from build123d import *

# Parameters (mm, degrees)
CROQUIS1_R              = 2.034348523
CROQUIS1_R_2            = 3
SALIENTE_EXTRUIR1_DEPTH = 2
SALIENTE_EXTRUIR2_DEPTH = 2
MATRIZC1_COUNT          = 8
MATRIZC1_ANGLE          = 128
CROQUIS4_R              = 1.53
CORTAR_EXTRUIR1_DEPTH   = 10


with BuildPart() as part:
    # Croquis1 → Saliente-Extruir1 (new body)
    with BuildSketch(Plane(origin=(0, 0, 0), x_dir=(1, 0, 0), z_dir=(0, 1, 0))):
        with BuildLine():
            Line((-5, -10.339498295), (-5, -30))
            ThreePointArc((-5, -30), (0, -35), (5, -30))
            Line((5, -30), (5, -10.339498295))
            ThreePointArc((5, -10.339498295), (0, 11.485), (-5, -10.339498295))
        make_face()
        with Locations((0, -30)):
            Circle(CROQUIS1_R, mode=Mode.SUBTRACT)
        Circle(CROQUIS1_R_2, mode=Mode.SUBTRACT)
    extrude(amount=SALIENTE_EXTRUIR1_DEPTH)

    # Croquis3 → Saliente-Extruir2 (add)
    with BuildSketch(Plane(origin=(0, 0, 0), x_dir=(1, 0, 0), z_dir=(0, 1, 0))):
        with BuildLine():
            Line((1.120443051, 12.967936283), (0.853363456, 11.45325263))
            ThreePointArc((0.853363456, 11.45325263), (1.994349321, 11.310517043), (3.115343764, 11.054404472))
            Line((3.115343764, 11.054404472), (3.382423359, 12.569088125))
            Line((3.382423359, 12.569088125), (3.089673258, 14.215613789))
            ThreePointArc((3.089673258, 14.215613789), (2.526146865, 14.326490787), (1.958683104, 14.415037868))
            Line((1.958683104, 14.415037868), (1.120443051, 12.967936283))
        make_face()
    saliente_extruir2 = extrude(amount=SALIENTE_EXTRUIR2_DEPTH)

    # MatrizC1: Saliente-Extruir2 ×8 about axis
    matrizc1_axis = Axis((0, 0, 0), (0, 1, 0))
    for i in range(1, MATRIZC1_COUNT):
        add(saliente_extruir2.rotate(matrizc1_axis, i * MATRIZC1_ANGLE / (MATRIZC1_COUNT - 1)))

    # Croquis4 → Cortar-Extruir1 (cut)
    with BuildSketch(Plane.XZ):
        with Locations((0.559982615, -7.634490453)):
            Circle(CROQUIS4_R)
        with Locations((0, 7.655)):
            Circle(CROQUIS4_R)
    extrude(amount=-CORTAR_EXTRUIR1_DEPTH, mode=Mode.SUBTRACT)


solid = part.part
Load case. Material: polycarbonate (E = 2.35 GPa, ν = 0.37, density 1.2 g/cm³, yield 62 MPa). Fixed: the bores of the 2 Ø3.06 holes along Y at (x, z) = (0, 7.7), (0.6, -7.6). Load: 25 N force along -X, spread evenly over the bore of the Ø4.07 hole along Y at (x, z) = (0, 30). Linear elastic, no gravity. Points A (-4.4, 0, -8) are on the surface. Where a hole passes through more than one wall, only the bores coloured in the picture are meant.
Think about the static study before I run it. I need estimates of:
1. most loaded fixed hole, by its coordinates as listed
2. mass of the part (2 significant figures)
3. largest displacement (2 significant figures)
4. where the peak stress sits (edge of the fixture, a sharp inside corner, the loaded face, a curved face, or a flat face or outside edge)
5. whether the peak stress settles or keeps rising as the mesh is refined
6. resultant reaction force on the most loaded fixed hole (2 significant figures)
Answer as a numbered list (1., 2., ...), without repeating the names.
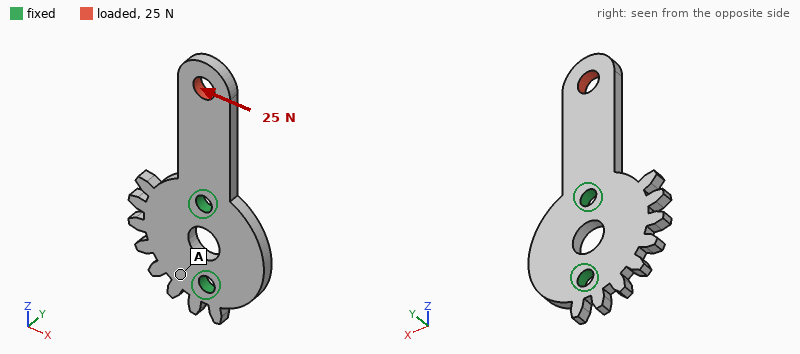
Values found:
1. (0, 7.7)
2. 1.5 g
3. 0.41 mm
4. a sharp inside corner
5. keeps rising
6. 46 N
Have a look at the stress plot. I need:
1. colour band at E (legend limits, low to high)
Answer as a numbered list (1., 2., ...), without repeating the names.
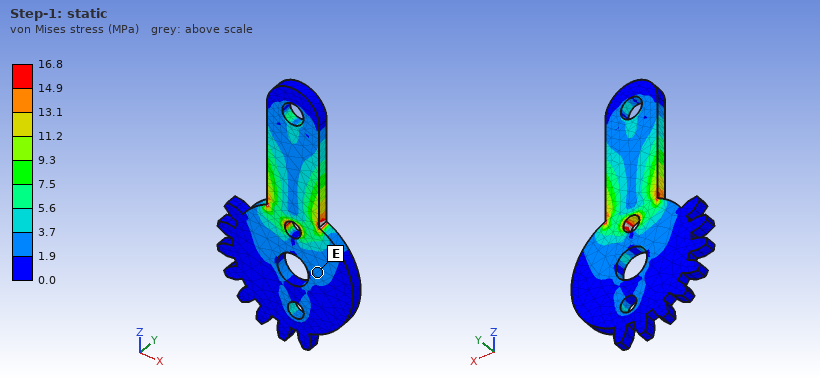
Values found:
1. 1.9 to 3.7 MPa
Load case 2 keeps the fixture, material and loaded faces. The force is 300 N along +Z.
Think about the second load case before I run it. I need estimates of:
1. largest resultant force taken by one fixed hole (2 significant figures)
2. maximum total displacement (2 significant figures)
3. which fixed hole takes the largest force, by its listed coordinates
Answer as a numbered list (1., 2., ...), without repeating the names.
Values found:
1. 270 N
2. 0.19 mm
3. (0, 7.7)
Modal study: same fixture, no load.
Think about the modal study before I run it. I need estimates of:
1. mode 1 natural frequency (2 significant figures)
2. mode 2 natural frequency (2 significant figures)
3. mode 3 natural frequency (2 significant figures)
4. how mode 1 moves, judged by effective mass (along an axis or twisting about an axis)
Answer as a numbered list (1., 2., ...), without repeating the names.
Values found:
1. 760 Hz
2. 2900 Hz
3. 3000 Hz
4. along Y
